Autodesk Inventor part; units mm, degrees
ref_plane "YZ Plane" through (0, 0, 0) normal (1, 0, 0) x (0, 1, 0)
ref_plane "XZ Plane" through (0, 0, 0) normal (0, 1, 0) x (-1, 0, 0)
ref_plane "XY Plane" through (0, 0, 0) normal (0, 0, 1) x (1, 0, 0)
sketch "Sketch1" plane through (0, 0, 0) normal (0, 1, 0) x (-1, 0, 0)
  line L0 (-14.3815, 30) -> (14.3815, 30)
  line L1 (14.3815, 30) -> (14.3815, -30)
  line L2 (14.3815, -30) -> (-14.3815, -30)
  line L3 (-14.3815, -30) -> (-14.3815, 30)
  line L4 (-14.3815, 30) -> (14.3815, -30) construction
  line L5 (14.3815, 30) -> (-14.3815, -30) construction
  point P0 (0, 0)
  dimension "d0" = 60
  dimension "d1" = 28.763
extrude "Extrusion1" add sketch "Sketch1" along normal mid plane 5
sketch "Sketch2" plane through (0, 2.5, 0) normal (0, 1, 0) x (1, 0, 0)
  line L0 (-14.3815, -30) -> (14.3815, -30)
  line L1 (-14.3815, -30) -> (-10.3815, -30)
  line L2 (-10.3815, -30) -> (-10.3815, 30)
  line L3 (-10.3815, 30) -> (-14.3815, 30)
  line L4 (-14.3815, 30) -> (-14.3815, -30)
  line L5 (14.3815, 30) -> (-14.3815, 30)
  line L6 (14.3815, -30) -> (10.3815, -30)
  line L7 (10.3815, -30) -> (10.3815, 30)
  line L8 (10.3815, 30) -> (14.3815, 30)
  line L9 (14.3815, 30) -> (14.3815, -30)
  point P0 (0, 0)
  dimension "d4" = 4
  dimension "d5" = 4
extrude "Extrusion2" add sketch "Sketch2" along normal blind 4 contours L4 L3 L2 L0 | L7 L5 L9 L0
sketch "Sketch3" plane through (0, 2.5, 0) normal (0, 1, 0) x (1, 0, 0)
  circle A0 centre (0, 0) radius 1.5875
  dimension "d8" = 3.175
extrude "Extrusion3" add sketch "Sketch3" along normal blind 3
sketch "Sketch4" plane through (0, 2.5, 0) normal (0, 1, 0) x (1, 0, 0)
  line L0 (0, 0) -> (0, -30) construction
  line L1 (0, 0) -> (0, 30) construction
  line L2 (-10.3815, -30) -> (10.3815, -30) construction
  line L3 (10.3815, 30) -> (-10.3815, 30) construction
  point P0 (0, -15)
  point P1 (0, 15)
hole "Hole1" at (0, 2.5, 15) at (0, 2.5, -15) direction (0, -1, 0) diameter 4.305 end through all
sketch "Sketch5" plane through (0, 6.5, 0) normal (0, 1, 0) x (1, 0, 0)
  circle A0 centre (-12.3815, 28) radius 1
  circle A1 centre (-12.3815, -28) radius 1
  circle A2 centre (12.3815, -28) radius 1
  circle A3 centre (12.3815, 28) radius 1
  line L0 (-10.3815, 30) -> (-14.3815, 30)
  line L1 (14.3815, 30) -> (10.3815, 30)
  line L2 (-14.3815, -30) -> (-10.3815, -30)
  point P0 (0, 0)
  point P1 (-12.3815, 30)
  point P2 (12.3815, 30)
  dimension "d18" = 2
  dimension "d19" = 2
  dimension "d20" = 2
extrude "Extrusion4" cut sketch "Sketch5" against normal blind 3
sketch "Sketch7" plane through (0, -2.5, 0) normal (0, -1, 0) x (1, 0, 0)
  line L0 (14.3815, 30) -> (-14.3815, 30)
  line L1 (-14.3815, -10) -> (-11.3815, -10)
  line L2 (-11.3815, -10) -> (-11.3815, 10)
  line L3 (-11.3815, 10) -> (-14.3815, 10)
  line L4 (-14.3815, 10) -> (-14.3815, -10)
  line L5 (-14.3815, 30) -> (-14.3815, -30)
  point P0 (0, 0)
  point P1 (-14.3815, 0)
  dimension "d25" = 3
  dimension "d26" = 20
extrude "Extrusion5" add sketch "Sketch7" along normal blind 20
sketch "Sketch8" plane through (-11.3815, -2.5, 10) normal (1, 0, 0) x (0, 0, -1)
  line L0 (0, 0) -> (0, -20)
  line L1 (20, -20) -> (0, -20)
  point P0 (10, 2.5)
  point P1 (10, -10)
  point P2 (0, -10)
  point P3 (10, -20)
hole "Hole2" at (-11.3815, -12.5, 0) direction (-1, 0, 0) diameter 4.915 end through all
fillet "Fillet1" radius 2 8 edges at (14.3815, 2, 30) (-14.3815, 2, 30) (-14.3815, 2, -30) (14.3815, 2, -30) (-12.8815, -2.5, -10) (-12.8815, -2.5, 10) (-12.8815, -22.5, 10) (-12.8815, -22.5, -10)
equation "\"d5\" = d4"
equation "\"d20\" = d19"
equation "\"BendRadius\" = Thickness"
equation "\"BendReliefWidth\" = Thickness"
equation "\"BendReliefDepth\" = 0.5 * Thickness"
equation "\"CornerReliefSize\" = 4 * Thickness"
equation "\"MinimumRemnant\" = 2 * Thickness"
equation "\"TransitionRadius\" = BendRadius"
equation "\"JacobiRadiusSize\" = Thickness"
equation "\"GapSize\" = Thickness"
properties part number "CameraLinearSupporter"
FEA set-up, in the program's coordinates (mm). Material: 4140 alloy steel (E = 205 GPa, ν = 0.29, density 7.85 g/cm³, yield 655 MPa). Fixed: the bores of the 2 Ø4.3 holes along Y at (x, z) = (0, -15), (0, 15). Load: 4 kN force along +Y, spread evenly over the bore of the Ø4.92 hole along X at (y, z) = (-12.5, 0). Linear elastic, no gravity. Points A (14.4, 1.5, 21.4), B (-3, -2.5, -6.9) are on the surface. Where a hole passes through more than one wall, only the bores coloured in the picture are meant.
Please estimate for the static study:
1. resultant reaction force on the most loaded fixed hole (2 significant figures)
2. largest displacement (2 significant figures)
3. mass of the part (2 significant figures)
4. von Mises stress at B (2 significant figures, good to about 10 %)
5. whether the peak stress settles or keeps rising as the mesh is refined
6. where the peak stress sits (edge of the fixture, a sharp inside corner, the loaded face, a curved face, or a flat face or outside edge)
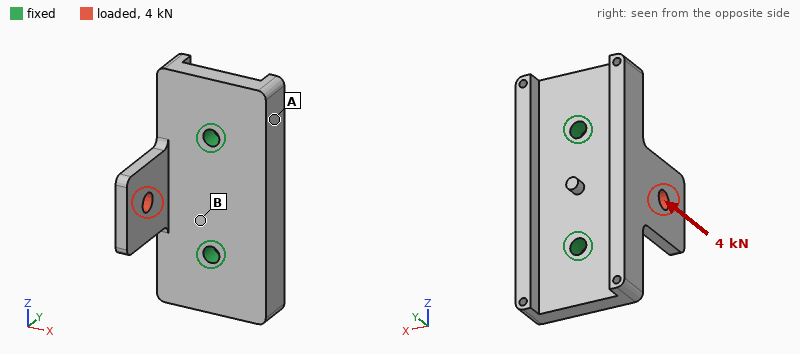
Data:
2.0 kN
0.10 mm
90 g
120 MPa
keeps rising
edge of the fixture
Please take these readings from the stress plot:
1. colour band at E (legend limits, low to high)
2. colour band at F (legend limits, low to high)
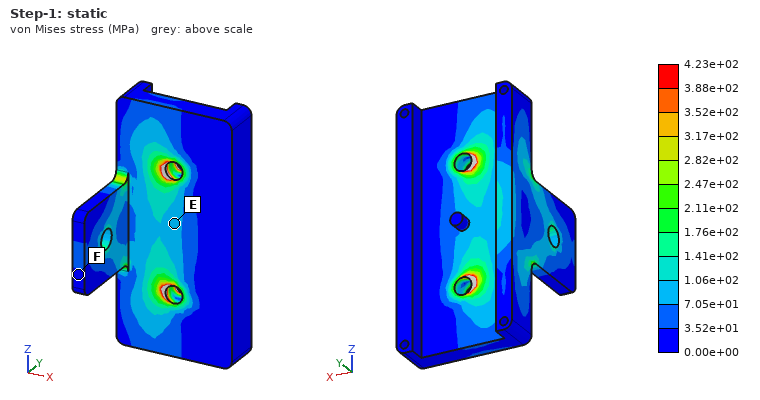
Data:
7.05e+01 to 1.06e+02 MPa
0.00e+00 to 3.52e+01 MPa
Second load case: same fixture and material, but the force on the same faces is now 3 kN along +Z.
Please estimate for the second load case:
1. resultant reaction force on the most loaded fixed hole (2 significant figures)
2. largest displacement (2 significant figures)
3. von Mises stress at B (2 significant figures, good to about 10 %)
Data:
2.3 kN
53 µm
72 MPa
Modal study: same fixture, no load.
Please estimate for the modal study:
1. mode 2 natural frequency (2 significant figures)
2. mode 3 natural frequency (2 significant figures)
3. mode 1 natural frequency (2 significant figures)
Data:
9900 Hz
11 kHz
4800 Hz
